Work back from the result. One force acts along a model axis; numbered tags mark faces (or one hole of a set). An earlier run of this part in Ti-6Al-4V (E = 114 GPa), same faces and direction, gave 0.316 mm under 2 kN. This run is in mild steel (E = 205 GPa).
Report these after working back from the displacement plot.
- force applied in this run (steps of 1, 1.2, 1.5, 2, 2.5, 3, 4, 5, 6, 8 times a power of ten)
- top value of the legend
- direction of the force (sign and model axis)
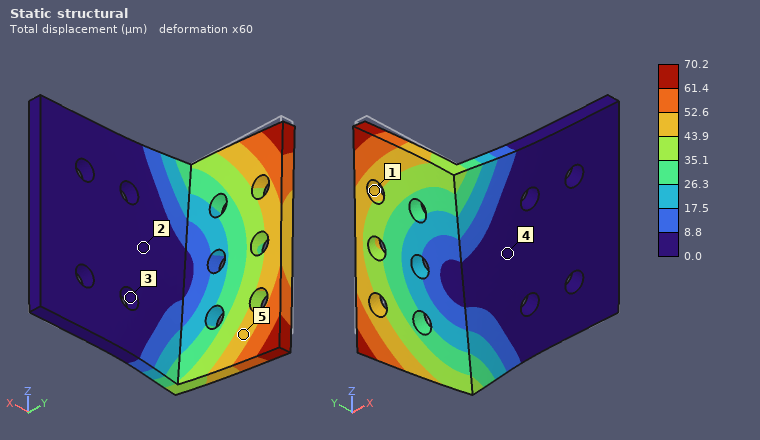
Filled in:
800 N
70.2 µm
-Z
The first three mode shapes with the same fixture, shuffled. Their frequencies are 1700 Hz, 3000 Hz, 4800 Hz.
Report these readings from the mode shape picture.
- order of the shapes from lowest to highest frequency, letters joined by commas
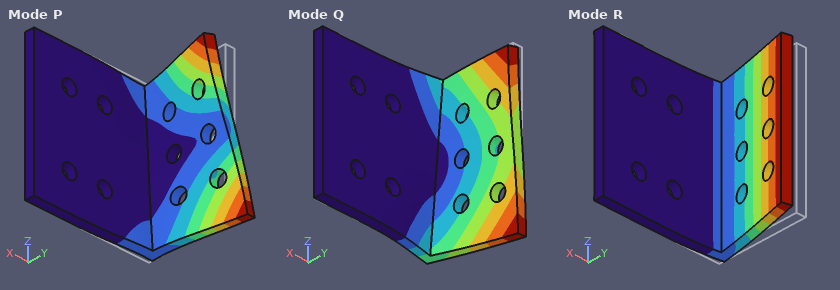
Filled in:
R, Q, P
